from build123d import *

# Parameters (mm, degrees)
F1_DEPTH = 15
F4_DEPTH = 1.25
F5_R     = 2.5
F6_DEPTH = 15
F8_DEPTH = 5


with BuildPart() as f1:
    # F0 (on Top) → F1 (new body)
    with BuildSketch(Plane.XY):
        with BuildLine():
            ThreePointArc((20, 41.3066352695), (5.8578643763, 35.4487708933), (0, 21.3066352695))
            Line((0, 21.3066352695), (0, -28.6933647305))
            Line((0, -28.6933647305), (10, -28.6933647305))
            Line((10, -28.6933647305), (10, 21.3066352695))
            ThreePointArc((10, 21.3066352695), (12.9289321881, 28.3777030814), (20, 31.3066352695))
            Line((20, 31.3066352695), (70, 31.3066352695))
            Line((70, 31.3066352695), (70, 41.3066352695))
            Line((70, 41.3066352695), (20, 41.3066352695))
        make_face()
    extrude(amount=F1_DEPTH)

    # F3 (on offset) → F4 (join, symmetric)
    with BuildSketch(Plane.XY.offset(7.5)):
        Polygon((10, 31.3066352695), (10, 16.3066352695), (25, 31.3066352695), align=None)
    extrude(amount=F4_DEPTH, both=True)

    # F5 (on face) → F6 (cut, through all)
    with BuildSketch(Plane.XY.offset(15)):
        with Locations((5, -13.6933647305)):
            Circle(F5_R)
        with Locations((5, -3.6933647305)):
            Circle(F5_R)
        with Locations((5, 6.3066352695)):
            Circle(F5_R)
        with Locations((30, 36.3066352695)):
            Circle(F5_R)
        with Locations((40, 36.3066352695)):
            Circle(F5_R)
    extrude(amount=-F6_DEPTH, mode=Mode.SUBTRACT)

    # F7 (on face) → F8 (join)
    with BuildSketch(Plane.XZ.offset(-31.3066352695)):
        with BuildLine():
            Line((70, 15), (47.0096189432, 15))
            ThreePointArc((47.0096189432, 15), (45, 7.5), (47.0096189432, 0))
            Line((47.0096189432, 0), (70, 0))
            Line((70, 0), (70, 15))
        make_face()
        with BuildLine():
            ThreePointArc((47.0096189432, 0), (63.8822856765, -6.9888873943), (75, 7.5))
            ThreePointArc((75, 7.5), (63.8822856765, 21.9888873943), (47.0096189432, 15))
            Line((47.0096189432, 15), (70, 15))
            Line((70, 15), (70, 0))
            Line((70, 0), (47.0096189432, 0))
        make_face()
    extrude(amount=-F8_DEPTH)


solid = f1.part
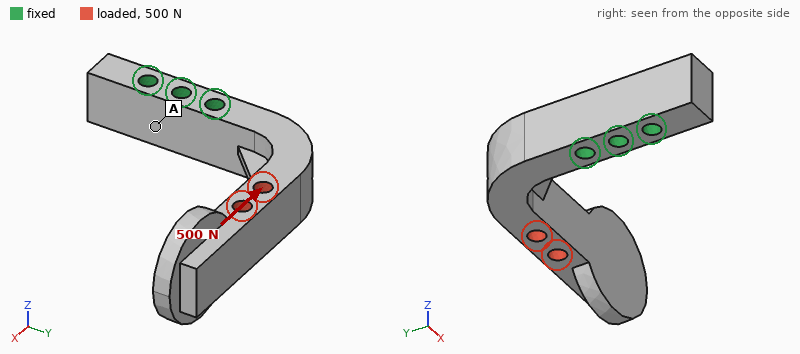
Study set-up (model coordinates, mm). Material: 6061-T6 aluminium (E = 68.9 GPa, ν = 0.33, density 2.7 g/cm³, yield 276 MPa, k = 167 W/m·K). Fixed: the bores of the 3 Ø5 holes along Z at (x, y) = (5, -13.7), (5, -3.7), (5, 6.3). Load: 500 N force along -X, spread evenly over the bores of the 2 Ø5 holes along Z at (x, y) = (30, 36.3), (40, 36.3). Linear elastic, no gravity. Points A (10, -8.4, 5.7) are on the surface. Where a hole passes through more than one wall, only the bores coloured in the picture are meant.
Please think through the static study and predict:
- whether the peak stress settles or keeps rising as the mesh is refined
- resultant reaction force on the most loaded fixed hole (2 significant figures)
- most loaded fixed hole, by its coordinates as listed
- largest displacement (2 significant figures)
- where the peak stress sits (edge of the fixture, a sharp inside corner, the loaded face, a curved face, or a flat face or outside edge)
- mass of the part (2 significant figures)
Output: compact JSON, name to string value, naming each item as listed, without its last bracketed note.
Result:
{"whether the peak stress settles or keeps rising as the mesh is refined": "keeps rising", "resultant reaction force on the most loaded fixed hole": "780 N", "most loaded fixed hole, by its coordinates as listed": "(5, 6.3)", "largest displacement": "0.19 mm", "where the peak stress sits": "edge of the fixture", "mass of the part": "51 g"}
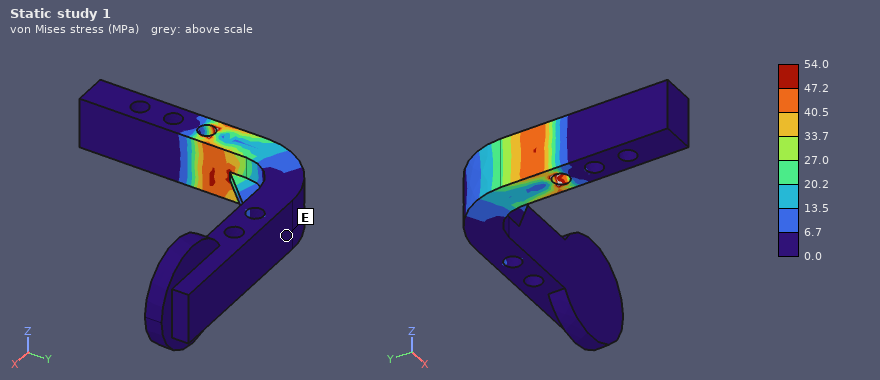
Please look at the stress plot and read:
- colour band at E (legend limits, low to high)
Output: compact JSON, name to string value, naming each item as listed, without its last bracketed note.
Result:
{"colour band at E": "0.0 to 6.7 MPa"}
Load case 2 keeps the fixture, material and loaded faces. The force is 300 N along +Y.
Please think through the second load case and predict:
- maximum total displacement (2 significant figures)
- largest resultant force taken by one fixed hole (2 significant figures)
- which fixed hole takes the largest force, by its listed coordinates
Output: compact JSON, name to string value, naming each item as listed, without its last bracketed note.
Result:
{"maximum total displacement": "0.21 mm", "largest resultant force taken by one fixed hole": "330 N", "which fixed hole takes the largest force, by its listed coordinates": "(5, 6.3)"}
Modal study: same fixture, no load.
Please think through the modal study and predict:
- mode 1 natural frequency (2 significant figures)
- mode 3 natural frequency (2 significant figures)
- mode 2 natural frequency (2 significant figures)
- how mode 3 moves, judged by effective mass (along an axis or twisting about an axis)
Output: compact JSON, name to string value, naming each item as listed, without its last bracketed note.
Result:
{"mode 1 natural frequency": "1100 Hz", "mode 3 natural frequency": "4100 Hz", "mode 2 natural frequency": "1100 Hz", "how mode 3 moves, judged by effective mass": "along X"}
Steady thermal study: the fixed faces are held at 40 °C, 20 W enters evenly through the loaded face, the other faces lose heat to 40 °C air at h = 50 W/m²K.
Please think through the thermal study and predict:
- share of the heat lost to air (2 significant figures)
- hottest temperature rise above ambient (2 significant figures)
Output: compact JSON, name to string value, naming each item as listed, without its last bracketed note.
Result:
{"share of the heat lost to air": "29 %", "hottest temperature rise above ambient": "30 K"}
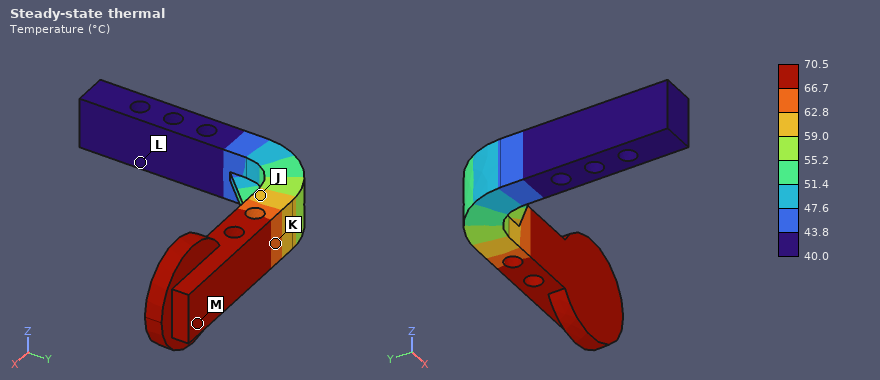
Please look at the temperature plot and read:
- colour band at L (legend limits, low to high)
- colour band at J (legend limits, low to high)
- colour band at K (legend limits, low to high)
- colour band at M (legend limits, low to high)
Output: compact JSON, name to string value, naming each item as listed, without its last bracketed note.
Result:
{"colour band at L": "40.0 to 43.8 °C", "colour band at J": "59.0 to 62.8 °C", "colour band at K": "62.8 to 66.7 °C", "colour band at M": "66.7 to 70.5 °C"}
